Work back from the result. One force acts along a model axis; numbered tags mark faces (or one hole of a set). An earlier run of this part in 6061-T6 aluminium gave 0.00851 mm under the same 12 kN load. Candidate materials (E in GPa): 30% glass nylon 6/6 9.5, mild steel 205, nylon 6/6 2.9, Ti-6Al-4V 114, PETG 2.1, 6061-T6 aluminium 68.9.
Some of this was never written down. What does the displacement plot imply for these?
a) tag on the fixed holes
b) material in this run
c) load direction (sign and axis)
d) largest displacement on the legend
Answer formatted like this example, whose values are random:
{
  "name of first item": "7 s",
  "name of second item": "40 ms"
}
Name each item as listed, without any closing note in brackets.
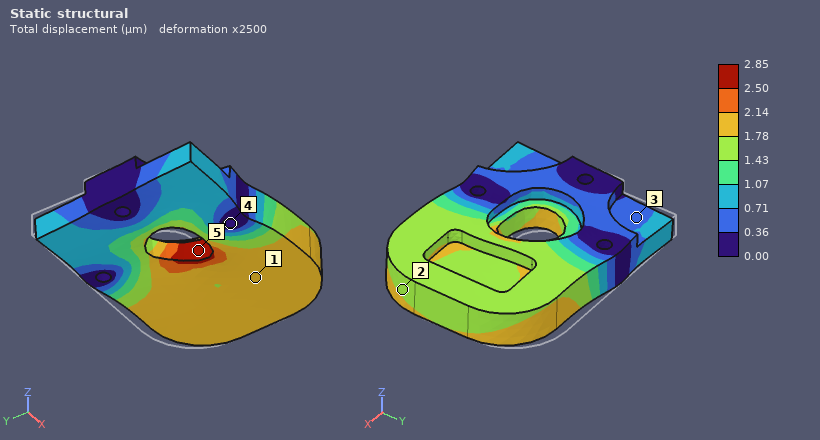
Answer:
{
  "tag on the fixed holes": "4",
  "material in this run": "mild steel",
  "load direction": "-Y",
  "largest displacement on the legend": "2.85 µm"
}
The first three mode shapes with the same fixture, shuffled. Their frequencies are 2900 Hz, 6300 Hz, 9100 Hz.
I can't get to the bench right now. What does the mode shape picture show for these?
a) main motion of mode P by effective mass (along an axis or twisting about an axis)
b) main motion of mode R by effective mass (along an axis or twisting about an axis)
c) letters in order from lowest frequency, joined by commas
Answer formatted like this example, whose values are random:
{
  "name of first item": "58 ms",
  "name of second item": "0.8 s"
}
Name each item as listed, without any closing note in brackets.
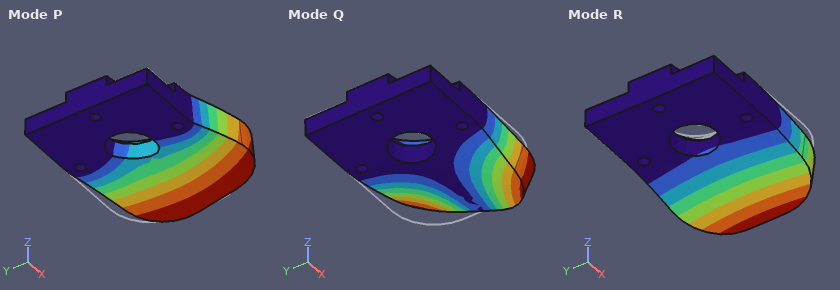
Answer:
{
  "main motion of mode P by effective mass": "along Y",
  "main motion of mode R by effective mass": "along Z",
  "letters in order from lowest frequency, joined by commas": "R, Q, P"
}
